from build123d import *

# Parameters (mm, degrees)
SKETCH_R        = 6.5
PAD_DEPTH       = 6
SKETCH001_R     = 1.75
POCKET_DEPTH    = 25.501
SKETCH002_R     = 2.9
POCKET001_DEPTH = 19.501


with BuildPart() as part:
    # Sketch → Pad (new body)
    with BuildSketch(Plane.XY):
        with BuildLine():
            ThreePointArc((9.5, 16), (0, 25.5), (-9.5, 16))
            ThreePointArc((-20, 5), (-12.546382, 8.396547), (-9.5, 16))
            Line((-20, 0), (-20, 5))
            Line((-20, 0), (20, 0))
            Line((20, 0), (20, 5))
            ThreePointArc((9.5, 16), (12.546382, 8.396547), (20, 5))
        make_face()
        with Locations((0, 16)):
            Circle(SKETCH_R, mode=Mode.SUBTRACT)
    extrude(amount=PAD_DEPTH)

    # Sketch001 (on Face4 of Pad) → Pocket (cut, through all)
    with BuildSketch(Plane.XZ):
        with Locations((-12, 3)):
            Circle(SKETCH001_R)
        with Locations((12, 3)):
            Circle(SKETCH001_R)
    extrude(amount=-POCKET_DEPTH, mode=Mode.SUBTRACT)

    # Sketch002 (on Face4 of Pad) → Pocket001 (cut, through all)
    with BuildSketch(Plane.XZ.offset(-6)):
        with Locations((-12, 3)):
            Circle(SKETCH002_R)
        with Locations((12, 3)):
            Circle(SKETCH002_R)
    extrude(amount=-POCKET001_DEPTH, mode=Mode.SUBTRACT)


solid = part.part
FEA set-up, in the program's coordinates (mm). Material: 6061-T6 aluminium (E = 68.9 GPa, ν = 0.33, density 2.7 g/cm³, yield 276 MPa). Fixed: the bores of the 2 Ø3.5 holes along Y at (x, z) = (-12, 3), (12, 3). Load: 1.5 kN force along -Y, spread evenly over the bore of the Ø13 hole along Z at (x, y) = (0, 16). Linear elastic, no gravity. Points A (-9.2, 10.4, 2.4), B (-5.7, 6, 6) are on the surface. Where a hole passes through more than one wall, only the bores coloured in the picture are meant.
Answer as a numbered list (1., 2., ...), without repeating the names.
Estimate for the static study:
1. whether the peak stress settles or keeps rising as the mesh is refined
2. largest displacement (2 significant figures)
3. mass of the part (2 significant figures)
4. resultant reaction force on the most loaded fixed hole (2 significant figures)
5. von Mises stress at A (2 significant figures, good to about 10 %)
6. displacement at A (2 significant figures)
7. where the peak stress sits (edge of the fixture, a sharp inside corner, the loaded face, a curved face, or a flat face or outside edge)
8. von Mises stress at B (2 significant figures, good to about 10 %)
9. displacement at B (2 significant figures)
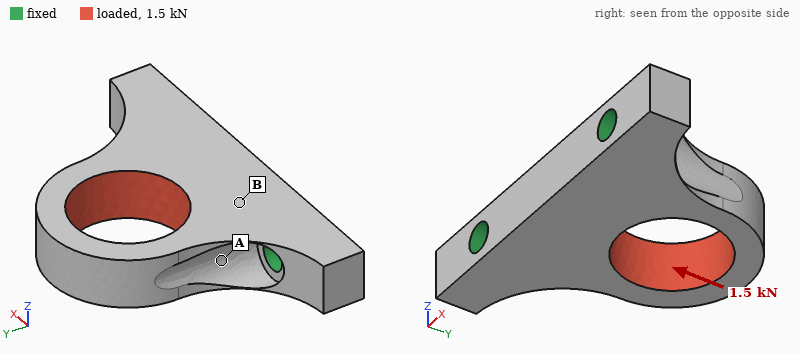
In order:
1. keeps rising
2. 14 µm
3. 6.8 g
4. 790 N
5. 32 MPa
6. 4.6 µm
7. edge of the fixture
8. 9.1 MPa
9. 3.5 µm
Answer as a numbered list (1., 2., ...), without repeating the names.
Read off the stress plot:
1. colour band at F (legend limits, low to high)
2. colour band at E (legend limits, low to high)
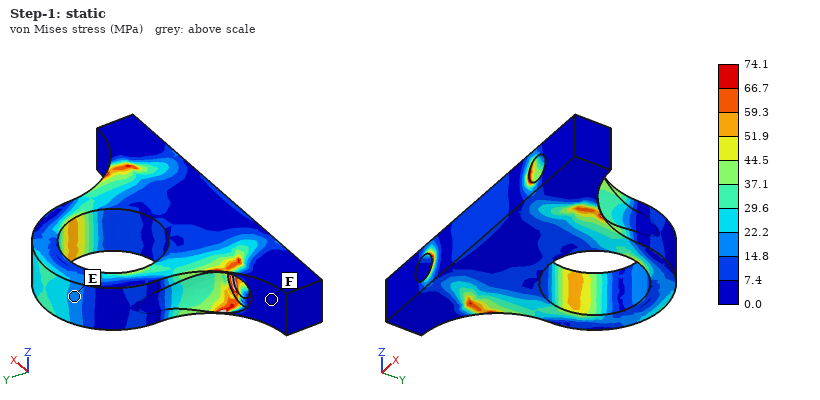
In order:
1. 0.0 to 7.4 MPa
2. 14.8 to 22.2 MPa
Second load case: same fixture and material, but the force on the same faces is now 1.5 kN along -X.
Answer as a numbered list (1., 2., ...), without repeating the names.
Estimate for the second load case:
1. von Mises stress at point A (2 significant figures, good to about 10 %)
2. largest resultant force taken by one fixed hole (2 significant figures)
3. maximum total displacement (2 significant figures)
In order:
1. 82 MPa
2. 1.2 kN
3. 65 µm
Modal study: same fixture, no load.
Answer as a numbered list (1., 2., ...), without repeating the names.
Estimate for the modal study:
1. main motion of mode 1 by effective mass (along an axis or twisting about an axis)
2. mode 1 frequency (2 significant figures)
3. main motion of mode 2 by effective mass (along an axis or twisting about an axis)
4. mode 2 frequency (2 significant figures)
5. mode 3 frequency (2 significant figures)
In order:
1. along Z
2. 9200 Hz
3. along X
4. 17 kHz
5. 21 kHz
